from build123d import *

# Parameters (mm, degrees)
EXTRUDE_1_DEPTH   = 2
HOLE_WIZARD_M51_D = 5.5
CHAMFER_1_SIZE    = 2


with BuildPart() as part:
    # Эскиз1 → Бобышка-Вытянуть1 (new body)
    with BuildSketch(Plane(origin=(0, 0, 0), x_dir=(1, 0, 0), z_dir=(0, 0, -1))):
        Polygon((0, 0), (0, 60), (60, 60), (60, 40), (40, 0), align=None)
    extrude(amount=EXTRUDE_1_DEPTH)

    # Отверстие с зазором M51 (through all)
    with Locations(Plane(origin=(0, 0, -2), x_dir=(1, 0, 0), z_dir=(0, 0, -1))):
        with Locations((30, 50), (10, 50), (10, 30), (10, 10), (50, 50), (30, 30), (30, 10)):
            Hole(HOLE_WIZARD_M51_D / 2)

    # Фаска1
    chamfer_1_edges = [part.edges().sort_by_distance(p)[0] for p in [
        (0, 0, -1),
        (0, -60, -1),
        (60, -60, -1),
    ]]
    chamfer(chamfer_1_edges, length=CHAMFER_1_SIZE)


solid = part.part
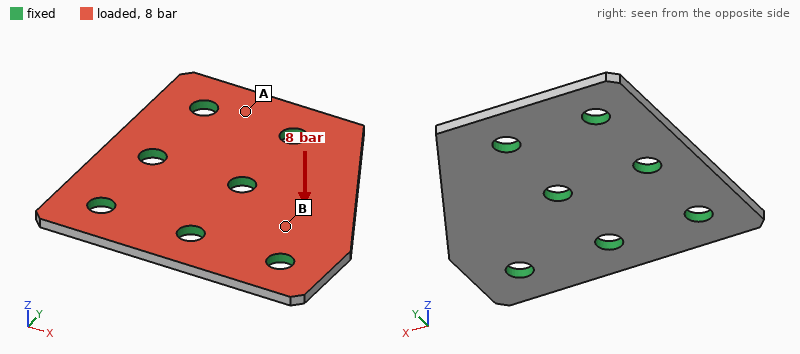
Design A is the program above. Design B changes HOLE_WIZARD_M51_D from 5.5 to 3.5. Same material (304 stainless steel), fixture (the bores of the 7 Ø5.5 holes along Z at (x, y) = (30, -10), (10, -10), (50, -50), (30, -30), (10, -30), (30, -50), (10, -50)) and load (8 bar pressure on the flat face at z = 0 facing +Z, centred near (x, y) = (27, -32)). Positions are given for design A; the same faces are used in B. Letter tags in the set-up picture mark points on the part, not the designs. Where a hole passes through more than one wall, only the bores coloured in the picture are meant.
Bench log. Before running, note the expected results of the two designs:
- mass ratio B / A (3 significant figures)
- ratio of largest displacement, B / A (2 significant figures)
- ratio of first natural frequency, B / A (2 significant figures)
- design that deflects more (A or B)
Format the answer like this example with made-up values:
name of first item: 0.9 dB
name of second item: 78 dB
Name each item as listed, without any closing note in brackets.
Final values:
mass ratio B / A: 1.03
ratio of largest displacement, B / A: 1.2
ratio of first natural frequency, B / A: 0.89
design that deflects more: B
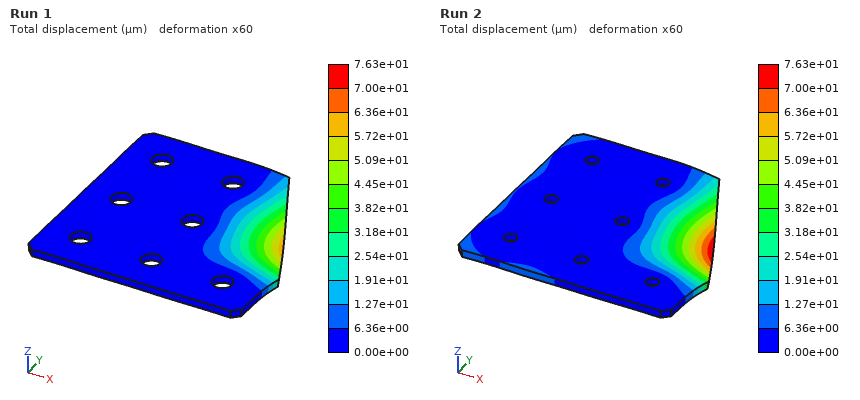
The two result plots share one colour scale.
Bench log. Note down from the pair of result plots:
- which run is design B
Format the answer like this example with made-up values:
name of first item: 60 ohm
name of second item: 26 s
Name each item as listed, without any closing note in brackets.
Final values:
which run is design B: Run 2
